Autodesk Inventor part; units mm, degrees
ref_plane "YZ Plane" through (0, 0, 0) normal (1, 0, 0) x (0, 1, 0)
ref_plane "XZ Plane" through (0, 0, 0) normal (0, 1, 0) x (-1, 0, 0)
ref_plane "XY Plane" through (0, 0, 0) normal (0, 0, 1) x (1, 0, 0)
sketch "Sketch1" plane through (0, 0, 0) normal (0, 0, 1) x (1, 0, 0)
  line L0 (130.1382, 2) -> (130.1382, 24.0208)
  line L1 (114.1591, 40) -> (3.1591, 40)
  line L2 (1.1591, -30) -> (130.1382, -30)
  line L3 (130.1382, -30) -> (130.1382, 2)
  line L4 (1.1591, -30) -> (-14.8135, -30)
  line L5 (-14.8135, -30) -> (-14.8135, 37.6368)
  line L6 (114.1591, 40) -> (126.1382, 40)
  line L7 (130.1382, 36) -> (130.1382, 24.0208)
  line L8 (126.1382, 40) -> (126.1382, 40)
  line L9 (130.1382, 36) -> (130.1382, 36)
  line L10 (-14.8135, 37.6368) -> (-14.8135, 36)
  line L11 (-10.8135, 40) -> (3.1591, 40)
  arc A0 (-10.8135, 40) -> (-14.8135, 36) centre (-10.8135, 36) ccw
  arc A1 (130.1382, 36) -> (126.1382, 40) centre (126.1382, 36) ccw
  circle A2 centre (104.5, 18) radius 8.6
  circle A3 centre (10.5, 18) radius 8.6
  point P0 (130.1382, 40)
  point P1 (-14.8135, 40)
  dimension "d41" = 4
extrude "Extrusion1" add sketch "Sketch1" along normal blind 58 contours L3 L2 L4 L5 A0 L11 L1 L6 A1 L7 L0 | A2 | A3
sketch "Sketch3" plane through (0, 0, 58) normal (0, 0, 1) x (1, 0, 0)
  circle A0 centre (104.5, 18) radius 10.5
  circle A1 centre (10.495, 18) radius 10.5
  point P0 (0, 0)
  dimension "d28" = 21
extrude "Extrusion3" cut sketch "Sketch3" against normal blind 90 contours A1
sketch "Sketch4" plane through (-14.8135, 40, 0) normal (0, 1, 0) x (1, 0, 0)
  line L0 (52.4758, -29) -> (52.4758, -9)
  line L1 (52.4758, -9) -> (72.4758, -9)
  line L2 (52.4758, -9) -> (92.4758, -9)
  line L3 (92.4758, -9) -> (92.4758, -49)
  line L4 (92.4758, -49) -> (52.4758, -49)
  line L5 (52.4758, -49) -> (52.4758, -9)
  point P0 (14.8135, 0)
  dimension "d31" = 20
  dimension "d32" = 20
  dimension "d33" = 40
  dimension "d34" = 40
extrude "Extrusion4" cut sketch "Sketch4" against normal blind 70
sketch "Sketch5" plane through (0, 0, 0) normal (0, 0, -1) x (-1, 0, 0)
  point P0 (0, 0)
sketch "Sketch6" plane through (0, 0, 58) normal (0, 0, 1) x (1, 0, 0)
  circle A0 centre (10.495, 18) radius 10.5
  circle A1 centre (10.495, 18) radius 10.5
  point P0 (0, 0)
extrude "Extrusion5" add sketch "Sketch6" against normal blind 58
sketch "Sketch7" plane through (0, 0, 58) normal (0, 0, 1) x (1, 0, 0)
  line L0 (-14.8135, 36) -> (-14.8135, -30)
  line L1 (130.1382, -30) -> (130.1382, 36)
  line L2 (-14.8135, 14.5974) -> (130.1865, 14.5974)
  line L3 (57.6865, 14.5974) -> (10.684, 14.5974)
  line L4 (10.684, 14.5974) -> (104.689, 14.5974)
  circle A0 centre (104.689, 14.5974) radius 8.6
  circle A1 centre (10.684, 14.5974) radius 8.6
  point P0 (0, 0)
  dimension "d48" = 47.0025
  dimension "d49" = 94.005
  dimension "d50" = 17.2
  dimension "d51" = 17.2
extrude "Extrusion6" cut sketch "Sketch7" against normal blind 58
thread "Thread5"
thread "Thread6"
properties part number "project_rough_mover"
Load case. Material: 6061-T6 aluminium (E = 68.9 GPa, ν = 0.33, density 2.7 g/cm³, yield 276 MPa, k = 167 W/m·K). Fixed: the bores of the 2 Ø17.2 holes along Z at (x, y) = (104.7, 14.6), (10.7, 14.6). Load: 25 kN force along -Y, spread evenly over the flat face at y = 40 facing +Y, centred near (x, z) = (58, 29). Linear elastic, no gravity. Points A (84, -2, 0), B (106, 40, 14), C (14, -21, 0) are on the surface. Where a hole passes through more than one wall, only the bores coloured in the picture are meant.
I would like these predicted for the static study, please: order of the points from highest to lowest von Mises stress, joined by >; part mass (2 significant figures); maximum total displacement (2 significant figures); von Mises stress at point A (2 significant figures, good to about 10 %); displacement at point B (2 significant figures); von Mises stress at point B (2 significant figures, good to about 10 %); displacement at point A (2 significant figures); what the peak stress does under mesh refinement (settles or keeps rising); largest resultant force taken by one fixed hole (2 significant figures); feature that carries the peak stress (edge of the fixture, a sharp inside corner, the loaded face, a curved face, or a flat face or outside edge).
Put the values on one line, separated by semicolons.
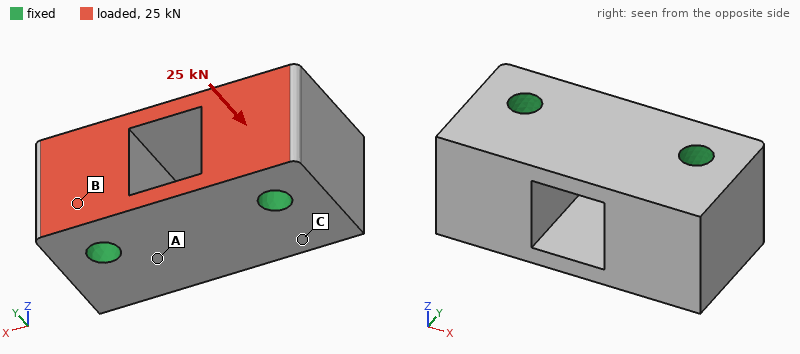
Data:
B > A > C; 1.2 kg; 4.3 µm; 2.9 MPa; 1.3 µm; 5.8 MPa; 1.5 µm; keeps rising; 13 kN; edge of the fixture
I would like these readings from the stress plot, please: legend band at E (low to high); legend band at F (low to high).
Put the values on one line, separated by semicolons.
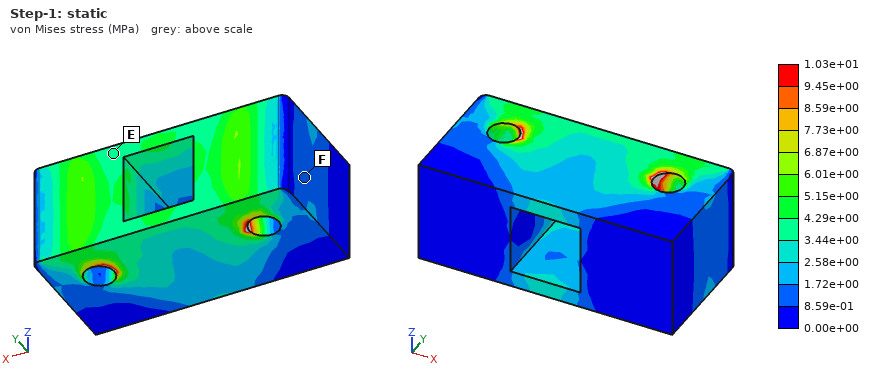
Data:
3.44e+00 to 4.29e+00 MPa; 8.59e-01 to 1.72e+00 MPa
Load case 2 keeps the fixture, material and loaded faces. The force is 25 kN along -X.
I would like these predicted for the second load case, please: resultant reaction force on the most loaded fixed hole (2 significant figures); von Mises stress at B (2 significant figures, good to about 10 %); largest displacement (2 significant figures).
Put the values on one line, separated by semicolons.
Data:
13 kN; 7.0 MPa; 7.8 µm
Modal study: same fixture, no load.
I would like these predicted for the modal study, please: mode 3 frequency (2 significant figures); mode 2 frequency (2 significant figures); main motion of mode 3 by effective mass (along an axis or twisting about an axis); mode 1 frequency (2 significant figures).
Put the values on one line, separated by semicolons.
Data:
12 kHz; 12 kHz; along X; 12 kHz
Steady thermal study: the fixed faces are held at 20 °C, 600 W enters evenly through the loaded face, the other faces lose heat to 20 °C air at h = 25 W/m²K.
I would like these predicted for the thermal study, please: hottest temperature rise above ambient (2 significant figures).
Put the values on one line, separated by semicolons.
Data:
19 K
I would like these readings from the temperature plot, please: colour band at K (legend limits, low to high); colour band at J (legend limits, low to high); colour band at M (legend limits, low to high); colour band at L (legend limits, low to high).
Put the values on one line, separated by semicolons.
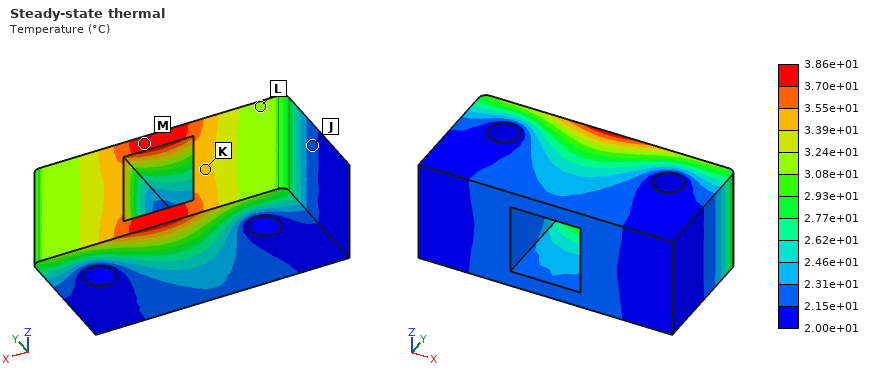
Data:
3.39e+01 to 3.55e+01 °C; 2.15e+01 to 2.31e+01 °C; 3.70e+01 to 3.86e+01 °C; 3.08e+01 to 3.24e+01 °C
